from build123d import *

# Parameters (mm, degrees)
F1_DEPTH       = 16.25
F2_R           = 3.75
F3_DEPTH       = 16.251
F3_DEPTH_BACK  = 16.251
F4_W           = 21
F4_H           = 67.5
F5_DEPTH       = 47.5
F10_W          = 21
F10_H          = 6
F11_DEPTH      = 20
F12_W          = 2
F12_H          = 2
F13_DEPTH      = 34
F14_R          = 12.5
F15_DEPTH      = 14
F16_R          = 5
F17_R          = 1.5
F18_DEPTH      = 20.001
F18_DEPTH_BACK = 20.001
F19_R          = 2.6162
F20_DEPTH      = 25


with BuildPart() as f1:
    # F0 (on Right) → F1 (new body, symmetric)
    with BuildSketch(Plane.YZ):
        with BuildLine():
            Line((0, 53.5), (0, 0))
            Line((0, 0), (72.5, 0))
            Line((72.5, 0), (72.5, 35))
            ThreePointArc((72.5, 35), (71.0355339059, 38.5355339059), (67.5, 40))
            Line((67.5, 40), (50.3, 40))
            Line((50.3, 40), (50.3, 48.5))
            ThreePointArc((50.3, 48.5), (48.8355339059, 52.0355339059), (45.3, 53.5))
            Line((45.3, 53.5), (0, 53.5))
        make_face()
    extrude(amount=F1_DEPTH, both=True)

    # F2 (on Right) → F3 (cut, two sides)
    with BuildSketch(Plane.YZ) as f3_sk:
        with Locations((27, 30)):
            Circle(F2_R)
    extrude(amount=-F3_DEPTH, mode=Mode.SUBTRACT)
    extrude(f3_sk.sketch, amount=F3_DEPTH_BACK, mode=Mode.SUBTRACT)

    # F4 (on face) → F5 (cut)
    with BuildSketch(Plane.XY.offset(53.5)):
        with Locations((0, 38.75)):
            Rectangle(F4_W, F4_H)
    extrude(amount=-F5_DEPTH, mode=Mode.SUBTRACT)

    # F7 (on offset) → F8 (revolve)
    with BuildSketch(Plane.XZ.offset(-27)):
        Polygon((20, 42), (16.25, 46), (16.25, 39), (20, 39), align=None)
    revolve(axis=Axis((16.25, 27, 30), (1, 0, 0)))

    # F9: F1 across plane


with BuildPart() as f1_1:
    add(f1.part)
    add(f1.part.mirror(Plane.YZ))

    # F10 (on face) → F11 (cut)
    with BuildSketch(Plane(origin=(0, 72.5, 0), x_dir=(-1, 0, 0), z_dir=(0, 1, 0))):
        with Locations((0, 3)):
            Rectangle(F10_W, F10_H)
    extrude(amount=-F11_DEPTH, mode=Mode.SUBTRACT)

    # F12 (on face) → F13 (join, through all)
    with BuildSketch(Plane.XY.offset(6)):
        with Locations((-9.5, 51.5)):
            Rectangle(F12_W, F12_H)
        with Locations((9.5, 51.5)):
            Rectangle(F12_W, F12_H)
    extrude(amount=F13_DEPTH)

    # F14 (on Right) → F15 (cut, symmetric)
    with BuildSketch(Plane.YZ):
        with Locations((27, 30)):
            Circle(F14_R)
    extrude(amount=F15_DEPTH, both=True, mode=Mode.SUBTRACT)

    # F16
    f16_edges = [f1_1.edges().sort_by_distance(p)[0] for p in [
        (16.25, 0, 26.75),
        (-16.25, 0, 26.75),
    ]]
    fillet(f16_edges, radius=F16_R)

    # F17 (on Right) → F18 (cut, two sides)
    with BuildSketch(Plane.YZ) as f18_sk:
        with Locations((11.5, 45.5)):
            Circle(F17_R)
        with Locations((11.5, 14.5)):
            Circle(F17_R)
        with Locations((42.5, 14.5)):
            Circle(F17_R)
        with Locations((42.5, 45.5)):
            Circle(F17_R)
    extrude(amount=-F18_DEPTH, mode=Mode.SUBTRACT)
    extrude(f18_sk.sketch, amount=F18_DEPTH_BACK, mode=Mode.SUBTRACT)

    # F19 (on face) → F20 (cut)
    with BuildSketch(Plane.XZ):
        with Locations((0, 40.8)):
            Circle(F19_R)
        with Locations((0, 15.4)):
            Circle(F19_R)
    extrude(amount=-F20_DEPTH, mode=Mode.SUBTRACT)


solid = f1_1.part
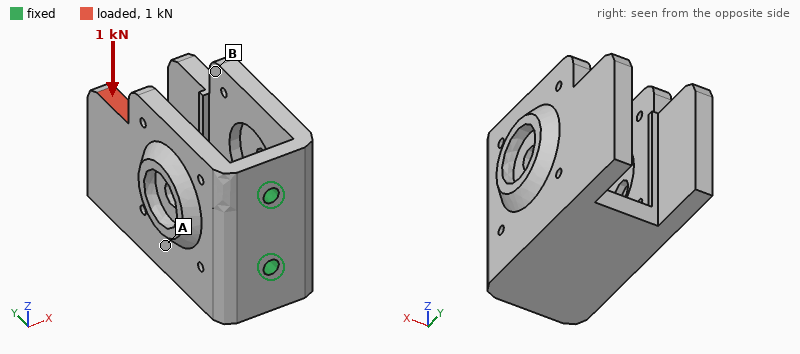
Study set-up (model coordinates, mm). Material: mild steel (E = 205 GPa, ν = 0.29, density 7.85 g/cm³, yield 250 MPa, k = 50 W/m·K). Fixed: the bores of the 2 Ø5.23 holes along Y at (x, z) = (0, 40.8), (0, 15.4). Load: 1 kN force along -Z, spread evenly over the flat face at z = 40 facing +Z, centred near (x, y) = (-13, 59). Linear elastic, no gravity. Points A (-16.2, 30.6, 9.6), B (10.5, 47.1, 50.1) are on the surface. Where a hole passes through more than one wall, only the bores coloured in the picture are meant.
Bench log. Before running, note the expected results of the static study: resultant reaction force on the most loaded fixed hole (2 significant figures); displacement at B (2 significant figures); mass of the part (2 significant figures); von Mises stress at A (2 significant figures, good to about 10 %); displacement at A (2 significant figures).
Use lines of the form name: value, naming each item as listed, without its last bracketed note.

resultant reaction force on the most loaded fixed hole: 1.9 kN
displacement at B: 33 µm
mass of the part: 400 g
von Mises stress at A: 16 MPa
displacement at A: 21 µm
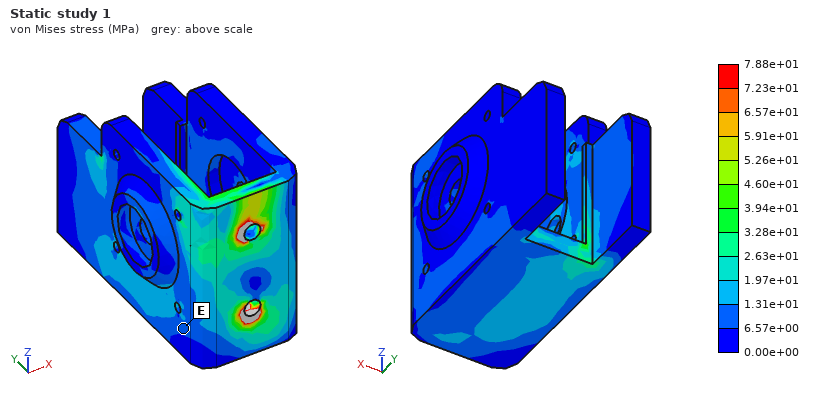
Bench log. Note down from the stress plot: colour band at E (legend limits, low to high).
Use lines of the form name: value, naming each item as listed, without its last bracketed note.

colour band at E: 6.57e+00 to 1.31e+01 MPa
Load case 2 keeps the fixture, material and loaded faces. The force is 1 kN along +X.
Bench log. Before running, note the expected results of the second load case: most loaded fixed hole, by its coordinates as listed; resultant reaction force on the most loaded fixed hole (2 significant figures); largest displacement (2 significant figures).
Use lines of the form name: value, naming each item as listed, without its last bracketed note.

most loaded fixed hole, by its coordinates as listed: (0, 40.8)
resultant reaction force on the most loaded fixed hole: 950 N
largest displacement: 0.37 mm
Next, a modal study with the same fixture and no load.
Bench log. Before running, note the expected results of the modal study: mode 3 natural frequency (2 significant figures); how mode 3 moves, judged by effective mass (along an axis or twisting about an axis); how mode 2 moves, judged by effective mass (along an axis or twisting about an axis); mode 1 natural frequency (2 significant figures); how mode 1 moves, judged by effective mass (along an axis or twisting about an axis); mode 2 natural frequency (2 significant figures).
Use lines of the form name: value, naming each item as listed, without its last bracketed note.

mode 3 natural frequency: 2800 Hz
how mode 3 moves, judged by effective mass: along Z
how mode 2 moves, judged by effective mass: along Z
mode 1 natural frequency: 980 Hz
how mode 1 moves, judged by effective mass: along X
mode 2 natural frequency: 2100 Hz
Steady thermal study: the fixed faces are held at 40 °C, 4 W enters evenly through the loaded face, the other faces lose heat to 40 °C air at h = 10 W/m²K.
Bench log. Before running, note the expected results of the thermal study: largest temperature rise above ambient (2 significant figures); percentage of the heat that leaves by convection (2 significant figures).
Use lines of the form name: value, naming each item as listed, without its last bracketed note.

largest temperature rise above ambient: 20 K
percentage of the heat that leaves by convection: 24 %
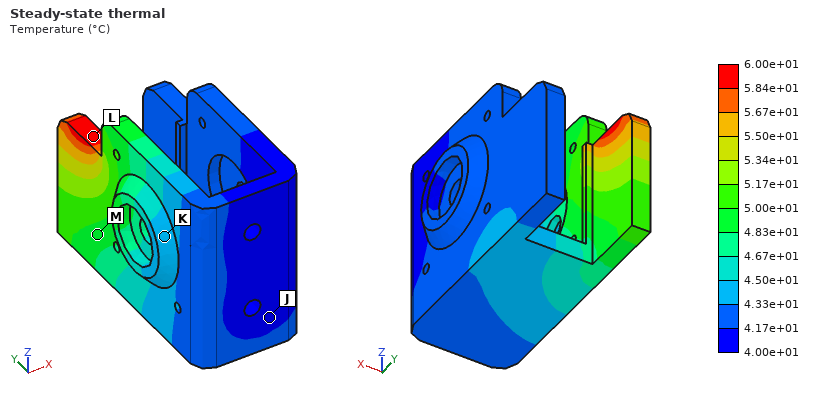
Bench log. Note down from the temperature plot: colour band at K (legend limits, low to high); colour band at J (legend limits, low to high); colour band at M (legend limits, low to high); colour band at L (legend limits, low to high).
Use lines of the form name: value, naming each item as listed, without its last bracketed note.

colour band at K: 4.33e+01 to 4.50e+01 °C
colour band at J: 4.00e+01 to 4.17e+01 °C
colour band at M: 4.83e+01 to 5.00e+01 °C
colour band at L: 5.84e+01 to 6.00e+01 °C
